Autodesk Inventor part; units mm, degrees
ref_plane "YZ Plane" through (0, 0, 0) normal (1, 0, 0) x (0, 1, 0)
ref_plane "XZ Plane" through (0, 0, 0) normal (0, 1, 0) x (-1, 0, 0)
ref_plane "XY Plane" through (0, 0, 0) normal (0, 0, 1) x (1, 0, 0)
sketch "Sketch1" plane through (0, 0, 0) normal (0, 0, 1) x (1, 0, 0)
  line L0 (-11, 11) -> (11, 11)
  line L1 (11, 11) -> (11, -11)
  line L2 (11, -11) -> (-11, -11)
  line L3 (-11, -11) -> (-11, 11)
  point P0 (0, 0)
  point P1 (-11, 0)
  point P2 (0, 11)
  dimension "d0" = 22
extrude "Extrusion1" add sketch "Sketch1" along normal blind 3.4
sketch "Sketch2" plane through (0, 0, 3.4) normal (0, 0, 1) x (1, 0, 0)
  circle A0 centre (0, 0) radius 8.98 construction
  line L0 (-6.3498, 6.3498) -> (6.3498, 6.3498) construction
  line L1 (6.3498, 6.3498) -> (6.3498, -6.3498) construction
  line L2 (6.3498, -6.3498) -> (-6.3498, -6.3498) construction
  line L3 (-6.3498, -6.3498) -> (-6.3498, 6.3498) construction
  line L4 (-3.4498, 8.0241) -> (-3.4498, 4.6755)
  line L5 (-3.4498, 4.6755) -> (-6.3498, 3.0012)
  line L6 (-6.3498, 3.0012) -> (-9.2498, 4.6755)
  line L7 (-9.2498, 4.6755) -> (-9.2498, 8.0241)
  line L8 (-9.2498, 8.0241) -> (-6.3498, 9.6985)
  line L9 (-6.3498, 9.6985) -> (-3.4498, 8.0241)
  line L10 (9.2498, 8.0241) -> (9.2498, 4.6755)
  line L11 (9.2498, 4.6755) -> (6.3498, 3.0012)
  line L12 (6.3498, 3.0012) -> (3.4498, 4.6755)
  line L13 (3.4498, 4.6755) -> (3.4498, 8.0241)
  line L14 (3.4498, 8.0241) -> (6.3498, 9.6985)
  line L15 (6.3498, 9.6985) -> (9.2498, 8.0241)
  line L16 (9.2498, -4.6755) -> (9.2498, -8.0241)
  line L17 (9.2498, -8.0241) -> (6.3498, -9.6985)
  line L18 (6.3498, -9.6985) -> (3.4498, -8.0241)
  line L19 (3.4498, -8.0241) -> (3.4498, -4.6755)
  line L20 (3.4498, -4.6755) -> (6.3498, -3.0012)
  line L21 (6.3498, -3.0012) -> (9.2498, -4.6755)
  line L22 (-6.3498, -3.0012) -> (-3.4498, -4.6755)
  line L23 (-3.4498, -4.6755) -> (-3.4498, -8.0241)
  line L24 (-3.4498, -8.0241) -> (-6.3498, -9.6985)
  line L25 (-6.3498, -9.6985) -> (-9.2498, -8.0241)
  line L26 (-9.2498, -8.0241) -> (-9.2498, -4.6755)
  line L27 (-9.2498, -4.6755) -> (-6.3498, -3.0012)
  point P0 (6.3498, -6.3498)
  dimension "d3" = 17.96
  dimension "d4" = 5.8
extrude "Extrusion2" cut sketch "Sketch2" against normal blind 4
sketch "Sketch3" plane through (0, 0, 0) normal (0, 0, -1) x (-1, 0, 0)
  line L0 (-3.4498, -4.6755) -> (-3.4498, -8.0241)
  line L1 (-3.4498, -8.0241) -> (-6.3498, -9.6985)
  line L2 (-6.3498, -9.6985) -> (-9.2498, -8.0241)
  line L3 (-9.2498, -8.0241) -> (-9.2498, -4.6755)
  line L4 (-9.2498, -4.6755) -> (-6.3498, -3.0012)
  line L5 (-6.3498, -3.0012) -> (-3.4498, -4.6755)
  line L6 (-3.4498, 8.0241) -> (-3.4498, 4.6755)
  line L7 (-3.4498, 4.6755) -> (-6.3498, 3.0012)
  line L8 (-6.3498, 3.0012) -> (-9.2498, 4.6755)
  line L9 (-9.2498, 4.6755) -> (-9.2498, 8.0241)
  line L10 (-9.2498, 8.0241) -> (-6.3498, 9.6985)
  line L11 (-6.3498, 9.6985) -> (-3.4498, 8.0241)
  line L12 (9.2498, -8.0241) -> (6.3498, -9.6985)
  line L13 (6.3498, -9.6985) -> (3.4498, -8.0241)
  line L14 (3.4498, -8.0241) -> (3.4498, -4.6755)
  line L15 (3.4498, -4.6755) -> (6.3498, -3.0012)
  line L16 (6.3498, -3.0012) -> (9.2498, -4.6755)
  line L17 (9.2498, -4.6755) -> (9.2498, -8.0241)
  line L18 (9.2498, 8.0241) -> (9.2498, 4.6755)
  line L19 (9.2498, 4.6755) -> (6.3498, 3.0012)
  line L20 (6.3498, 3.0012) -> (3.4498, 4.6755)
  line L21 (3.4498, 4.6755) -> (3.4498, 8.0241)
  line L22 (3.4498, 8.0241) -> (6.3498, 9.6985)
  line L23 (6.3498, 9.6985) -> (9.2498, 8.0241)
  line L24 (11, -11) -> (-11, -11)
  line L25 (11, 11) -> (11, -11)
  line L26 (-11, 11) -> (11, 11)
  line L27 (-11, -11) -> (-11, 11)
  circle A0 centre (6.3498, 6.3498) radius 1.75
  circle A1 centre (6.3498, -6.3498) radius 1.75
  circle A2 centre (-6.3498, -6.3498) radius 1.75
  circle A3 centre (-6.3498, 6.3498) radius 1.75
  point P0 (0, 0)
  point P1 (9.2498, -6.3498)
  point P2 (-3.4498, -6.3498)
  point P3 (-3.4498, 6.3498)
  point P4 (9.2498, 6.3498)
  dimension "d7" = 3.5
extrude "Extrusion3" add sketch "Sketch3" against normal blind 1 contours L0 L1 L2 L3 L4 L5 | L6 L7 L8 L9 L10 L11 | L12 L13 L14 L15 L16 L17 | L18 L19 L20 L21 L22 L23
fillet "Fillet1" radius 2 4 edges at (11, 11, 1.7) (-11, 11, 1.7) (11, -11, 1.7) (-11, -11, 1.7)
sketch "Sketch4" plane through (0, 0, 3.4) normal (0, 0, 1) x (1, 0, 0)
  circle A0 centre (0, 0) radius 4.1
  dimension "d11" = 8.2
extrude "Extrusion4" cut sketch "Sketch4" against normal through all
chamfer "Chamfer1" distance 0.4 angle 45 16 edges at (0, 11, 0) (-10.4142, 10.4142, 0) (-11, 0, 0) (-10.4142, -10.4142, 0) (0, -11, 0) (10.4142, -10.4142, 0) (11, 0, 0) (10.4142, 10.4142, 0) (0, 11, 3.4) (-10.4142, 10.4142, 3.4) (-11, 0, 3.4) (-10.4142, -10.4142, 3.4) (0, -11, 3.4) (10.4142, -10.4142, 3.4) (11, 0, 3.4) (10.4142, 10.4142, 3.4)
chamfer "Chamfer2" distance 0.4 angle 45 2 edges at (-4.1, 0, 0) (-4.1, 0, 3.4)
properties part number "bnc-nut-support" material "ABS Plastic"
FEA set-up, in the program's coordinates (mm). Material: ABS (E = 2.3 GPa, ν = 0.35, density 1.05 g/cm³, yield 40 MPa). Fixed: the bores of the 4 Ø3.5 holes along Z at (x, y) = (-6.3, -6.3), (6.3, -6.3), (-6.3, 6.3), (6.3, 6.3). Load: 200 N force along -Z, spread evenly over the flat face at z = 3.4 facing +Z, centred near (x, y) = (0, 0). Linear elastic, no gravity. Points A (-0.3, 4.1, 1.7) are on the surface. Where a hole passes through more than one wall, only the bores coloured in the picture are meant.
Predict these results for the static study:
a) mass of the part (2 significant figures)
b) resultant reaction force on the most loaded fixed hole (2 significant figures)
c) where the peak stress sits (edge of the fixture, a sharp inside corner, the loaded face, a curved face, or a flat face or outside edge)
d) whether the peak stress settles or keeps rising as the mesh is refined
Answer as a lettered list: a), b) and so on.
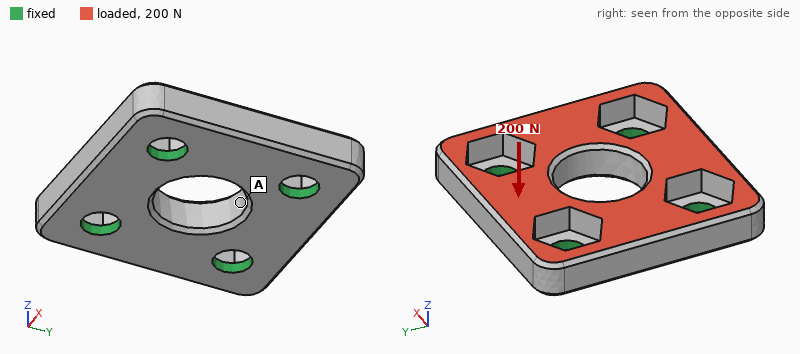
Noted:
a) 1.2 g
b) 51 N
c) edge of the fixture
d) keeps rising
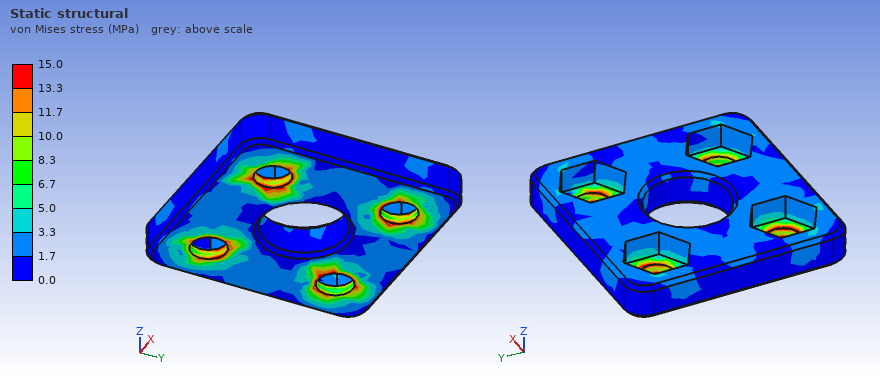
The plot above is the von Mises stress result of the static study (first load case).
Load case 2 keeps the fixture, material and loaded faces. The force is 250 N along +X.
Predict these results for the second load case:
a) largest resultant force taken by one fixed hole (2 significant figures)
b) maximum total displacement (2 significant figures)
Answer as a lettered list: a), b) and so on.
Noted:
a) 67 N
b) 50 µm
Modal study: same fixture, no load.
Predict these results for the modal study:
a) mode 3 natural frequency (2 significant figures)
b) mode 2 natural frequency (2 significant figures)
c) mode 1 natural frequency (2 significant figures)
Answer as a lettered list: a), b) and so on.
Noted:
a) 14 kHz
b) 14 kHz
c) 12 kHz
